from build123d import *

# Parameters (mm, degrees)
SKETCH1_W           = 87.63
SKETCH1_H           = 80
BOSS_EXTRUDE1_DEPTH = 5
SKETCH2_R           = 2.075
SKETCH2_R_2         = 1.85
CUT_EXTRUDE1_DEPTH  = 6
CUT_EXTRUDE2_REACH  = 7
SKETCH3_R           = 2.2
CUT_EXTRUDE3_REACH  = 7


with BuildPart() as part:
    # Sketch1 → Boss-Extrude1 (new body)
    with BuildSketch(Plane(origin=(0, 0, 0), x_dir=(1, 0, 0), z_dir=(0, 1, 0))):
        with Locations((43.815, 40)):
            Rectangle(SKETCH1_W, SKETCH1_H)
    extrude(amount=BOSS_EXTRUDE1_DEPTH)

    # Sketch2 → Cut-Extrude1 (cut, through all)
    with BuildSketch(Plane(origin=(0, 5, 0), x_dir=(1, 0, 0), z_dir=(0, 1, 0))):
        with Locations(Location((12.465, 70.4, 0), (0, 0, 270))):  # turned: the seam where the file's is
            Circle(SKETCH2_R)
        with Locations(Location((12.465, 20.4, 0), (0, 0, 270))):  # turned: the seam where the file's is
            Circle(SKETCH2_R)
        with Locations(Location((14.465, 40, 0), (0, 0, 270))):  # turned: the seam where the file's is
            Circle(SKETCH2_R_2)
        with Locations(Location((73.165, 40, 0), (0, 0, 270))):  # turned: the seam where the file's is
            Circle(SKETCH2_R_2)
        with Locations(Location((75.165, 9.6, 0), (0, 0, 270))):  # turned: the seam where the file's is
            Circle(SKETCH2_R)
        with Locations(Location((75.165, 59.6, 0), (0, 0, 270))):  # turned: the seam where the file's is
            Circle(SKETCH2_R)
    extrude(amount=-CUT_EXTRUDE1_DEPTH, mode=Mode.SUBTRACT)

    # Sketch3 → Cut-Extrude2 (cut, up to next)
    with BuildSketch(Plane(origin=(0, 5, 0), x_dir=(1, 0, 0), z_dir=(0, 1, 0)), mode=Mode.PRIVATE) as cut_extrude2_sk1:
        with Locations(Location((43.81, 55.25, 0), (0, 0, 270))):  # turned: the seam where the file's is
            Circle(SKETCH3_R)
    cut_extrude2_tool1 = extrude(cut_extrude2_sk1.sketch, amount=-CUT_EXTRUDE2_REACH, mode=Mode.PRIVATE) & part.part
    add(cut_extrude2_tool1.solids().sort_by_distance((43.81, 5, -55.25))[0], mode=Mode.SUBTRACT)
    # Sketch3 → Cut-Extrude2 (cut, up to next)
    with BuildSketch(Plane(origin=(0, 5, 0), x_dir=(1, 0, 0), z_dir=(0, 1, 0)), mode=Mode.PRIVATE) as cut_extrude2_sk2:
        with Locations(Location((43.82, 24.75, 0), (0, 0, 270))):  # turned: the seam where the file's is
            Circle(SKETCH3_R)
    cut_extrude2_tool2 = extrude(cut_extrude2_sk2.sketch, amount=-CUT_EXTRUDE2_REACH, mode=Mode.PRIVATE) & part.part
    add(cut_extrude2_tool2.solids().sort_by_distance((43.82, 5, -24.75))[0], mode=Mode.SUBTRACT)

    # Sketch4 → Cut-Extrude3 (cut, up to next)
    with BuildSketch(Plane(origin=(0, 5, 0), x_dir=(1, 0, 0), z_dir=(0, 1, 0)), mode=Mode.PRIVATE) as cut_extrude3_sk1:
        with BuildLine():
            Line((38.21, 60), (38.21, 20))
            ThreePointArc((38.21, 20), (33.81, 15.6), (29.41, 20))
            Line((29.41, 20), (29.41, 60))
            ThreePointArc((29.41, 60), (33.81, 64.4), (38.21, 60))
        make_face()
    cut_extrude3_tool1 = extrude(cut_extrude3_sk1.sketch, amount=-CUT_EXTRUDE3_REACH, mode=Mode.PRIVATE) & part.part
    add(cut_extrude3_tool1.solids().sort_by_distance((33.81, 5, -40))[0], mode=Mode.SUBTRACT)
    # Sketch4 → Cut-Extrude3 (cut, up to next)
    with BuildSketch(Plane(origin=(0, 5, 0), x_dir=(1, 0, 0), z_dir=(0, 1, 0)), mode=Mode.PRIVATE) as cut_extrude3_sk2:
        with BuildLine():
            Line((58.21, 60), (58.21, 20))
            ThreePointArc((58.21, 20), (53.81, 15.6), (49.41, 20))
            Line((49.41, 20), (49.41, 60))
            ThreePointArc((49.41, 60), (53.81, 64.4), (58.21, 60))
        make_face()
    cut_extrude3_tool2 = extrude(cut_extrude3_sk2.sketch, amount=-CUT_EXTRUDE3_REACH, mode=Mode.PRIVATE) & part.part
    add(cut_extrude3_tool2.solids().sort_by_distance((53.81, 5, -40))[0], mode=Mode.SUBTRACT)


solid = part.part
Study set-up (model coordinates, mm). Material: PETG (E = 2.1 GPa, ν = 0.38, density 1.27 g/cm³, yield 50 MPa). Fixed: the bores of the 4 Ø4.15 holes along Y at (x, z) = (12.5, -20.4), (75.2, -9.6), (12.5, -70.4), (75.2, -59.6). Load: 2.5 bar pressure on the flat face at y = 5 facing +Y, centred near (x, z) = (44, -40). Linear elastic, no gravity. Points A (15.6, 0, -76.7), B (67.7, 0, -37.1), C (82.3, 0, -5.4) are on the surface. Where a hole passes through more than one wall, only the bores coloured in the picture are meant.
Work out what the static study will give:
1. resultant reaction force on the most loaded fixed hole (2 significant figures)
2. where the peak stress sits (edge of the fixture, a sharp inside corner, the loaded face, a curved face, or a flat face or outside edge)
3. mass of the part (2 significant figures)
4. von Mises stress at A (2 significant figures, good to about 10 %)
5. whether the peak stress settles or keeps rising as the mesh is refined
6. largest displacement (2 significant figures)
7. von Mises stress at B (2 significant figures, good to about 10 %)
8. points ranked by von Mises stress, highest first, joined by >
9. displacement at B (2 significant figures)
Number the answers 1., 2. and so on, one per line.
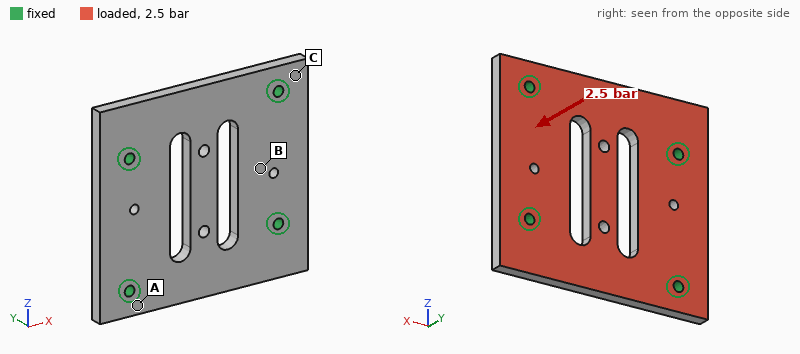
1. 430 N
2. edge of the fixture
3. 39 g
4. 11 MPa
5. keeps rising
6. 1.2 mm
7. 5.8 MPa
8. A > B > C
9. 0.33 mm
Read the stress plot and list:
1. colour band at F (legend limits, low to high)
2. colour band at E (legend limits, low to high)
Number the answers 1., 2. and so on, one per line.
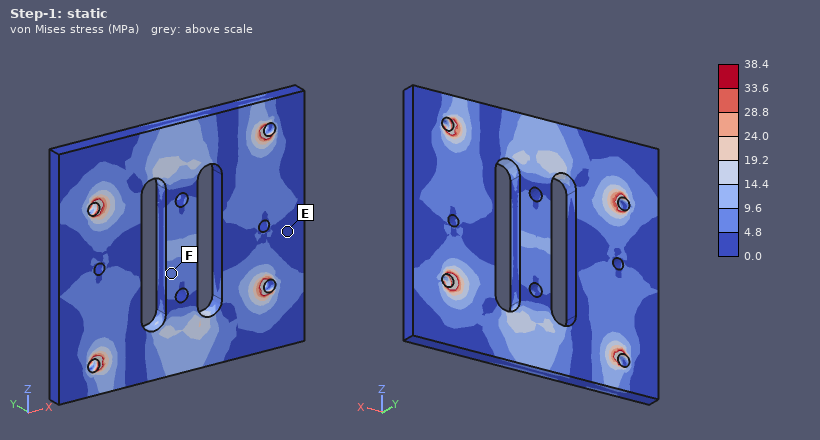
1. 4.8 to 9.6 MPa
2. 0.0 to 4.8 MPa
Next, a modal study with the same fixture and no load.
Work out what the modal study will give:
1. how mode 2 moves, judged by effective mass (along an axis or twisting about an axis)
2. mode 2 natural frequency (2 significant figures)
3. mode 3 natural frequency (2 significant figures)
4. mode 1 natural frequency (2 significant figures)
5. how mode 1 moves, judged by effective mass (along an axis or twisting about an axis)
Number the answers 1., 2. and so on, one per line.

1. twisting about X
2. 1500 Hz
3. 1700 Hz
4. 1100 Hz
5. along Y
